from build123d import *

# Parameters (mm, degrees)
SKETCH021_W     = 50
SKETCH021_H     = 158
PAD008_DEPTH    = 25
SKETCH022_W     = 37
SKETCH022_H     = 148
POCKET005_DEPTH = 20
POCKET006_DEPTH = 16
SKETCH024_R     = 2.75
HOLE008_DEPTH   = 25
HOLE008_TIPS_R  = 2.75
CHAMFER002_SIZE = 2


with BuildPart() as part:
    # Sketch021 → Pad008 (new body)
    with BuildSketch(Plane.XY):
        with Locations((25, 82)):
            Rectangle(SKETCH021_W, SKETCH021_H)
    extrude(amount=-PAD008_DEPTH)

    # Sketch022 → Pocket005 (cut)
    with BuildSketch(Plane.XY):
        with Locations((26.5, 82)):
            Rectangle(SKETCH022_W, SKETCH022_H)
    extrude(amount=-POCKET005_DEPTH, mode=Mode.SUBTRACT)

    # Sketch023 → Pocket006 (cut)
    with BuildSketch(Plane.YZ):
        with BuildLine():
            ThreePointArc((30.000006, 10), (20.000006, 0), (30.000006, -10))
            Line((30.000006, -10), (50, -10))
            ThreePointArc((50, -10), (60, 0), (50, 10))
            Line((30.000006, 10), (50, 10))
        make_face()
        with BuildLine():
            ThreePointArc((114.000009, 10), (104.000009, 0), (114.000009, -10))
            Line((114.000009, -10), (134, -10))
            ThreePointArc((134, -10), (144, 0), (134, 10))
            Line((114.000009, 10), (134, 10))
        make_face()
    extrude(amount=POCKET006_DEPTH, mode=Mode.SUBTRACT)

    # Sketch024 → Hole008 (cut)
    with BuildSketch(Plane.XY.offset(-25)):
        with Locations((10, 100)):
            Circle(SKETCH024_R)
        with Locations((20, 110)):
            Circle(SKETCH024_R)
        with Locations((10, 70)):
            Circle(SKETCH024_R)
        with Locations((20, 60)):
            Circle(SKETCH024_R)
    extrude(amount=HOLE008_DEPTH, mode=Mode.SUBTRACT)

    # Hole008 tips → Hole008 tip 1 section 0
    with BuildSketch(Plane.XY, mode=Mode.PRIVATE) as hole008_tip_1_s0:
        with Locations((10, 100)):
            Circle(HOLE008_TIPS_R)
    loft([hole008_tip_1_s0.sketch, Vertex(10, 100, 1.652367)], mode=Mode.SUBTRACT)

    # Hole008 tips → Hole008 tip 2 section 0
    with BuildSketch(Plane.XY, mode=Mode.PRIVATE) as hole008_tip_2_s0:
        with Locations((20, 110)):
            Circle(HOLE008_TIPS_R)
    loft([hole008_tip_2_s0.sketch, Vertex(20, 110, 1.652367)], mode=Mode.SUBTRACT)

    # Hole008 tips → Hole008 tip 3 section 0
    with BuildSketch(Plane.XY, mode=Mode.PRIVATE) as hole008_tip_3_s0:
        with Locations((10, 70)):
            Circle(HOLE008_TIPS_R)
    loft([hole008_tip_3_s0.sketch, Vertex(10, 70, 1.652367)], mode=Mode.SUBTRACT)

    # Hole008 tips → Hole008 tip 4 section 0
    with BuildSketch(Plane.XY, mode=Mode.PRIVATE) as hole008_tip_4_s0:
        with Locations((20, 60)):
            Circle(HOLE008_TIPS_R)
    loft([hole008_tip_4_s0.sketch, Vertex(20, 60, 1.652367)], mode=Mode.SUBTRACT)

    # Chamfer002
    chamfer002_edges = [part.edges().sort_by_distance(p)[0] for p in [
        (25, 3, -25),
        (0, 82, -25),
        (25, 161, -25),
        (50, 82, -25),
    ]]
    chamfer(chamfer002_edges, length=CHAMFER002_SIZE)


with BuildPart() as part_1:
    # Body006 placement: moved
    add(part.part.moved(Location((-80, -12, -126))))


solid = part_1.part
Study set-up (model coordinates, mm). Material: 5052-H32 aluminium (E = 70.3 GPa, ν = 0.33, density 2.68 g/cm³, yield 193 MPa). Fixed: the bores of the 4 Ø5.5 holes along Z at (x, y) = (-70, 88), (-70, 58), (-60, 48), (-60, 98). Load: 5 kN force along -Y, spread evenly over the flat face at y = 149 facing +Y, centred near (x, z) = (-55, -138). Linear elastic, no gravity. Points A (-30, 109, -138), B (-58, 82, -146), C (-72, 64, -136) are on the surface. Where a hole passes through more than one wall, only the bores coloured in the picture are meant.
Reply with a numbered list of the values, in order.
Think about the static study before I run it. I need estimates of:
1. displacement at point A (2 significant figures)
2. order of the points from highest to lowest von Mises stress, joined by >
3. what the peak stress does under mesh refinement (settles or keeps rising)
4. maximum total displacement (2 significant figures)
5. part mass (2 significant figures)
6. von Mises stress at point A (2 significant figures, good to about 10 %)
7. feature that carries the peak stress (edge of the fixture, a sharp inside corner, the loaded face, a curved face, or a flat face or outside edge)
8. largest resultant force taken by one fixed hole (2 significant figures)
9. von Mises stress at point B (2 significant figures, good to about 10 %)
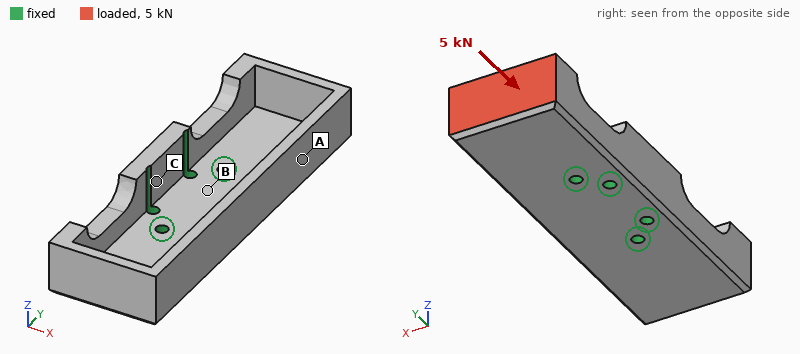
1. 0.062 mm
2. A > B > C
3. keeps rising
4. 0.20 mm
5. 220 g
6. 22 MPa
7. edge of the fixture
8. 2.0 kN
9. 15 MPa
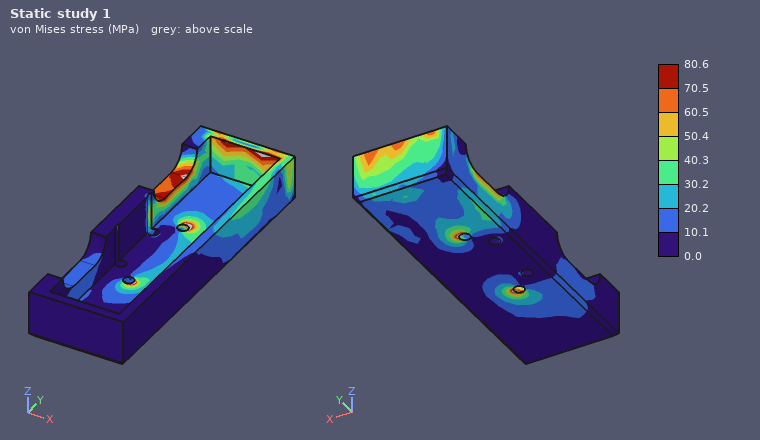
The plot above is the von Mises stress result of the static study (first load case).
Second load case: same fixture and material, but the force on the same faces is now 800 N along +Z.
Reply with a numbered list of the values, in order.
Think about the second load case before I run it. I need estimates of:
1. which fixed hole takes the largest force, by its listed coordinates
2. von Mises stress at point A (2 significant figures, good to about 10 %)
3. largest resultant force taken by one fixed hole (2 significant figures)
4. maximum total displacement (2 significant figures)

1. (-60, 98)
2. 12 MPa
3. 1.5 kN
4. 0.19 mm
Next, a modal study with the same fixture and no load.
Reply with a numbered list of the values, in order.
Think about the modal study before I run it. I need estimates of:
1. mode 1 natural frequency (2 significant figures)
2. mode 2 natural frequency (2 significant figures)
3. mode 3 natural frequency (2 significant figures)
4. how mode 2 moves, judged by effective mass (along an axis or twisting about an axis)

1. 1500 Hz
2. 1800 Hz
3. 2600 Hz
4. along Z
